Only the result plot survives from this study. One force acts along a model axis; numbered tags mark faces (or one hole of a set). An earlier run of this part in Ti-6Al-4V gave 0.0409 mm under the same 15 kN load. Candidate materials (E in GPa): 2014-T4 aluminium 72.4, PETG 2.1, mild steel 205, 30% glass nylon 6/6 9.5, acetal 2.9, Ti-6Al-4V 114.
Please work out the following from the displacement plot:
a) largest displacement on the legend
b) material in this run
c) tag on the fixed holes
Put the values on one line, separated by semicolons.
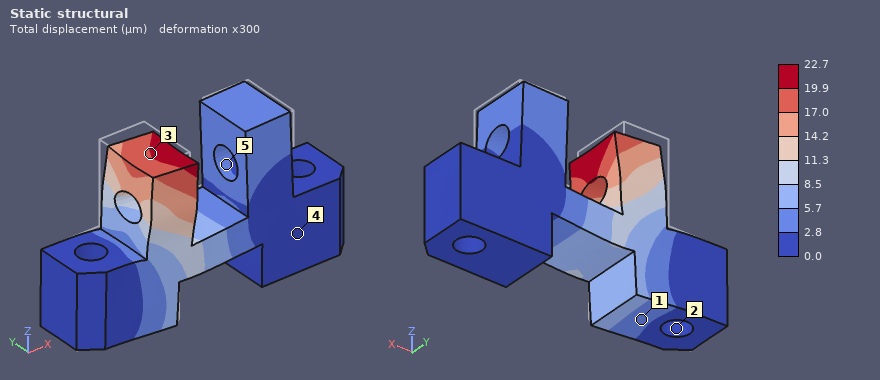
22.7 µm; mild steel; 2
